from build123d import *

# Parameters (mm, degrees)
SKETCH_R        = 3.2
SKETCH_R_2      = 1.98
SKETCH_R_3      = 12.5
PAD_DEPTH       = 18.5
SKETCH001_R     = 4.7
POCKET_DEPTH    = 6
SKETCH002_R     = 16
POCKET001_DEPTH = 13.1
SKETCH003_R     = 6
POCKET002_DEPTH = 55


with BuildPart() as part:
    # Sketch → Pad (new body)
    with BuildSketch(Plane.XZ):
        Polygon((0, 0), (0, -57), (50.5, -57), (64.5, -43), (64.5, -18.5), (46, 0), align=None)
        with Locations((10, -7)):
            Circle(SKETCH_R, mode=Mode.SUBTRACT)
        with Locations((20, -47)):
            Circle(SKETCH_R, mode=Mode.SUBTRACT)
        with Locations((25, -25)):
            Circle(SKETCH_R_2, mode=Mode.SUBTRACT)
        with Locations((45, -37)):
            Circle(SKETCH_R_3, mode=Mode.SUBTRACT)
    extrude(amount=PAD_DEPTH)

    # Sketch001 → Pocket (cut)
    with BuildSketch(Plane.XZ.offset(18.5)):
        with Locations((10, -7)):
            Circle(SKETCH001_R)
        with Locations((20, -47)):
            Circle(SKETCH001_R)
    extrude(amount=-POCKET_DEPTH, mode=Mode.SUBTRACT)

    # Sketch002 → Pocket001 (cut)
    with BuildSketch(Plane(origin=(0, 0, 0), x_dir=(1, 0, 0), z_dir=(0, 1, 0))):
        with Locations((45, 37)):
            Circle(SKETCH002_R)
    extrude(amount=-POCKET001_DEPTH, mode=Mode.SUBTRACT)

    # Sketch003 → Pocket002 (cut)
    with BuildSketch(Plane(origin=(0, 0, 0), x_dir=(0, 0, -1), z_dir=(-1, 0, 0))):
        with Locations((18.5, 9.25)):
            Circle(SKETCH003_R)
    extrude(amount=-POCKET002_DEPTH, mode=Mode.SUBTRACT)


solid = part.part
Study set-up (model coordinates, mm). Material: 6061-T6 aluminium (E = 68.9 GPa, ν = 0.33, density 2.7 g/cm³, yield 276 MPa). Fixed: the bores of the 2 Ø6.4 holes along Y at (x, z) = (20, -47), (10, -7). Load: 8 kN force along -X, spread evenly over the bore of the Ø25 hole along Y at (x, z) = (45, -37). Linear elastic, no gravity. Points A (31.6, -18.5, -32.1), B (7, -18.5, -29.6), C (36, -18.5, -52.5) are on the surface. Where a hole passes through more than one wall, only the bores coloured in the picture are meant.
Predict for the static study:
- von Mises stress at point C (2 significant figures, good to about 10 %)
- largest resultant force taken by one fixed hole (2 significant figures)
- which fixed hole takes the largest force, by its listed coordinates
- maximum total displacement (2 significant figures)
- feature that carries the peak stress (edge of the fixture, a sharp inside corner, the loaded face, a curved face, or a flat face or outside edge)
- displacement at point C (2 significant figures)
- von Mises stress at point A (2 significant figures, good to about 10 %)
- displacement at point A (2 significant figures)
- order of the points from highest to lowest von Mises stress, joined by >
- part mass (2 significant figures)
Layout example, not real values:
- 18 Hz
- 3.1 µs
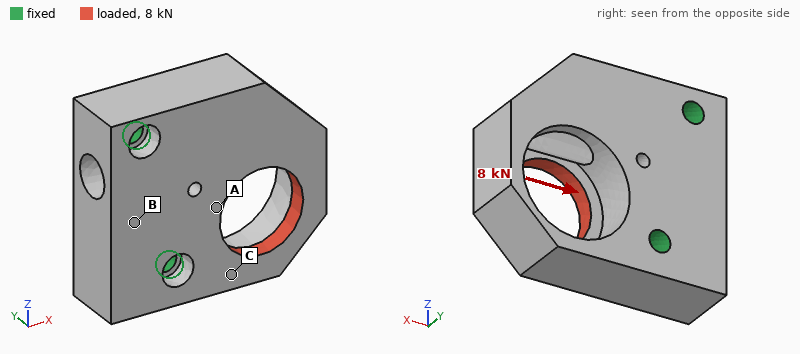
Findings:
- 57 MPa
- 5.8 kN
- (20, -47)
- 86 µm
- edge of the fixture
- 29 µm
- 31 MPa
- 22 µm
- C > A > B
- 110 g
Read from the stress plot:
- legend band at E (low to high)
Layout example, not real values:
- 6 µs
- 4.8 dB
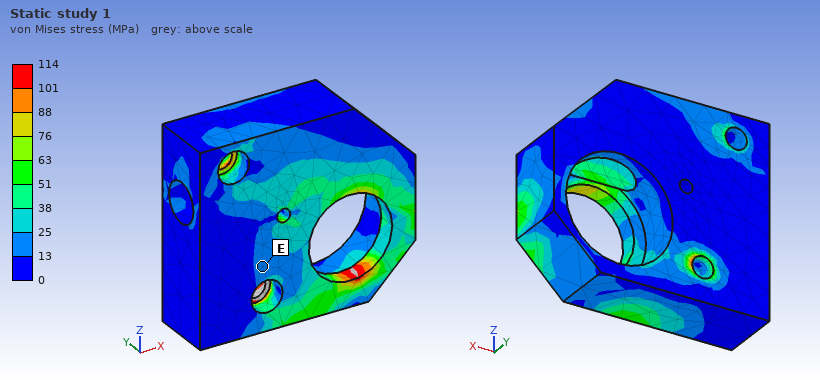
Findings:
- 13 to 25 MPa
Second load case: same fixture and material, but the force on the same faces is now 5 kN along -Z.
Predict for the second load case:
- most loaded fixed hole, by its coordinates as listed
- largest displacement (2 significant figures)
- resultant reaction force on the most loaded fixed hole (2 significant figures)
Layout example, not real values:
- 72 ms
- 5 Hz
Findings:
- (20, -47)
- 56 µm
- 5.1 kN
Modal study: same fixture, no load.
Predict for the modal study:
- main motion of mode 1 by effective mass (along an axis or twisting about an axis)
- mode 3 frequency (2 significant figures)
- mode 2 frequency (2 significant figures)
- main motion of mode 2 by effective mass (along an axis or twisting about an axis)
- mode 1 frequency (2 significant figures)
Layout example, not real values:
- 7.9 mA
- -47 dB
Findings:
- along Y
- 11 kHz
- 8600 Hz
- along Z
- 4800 Hz
